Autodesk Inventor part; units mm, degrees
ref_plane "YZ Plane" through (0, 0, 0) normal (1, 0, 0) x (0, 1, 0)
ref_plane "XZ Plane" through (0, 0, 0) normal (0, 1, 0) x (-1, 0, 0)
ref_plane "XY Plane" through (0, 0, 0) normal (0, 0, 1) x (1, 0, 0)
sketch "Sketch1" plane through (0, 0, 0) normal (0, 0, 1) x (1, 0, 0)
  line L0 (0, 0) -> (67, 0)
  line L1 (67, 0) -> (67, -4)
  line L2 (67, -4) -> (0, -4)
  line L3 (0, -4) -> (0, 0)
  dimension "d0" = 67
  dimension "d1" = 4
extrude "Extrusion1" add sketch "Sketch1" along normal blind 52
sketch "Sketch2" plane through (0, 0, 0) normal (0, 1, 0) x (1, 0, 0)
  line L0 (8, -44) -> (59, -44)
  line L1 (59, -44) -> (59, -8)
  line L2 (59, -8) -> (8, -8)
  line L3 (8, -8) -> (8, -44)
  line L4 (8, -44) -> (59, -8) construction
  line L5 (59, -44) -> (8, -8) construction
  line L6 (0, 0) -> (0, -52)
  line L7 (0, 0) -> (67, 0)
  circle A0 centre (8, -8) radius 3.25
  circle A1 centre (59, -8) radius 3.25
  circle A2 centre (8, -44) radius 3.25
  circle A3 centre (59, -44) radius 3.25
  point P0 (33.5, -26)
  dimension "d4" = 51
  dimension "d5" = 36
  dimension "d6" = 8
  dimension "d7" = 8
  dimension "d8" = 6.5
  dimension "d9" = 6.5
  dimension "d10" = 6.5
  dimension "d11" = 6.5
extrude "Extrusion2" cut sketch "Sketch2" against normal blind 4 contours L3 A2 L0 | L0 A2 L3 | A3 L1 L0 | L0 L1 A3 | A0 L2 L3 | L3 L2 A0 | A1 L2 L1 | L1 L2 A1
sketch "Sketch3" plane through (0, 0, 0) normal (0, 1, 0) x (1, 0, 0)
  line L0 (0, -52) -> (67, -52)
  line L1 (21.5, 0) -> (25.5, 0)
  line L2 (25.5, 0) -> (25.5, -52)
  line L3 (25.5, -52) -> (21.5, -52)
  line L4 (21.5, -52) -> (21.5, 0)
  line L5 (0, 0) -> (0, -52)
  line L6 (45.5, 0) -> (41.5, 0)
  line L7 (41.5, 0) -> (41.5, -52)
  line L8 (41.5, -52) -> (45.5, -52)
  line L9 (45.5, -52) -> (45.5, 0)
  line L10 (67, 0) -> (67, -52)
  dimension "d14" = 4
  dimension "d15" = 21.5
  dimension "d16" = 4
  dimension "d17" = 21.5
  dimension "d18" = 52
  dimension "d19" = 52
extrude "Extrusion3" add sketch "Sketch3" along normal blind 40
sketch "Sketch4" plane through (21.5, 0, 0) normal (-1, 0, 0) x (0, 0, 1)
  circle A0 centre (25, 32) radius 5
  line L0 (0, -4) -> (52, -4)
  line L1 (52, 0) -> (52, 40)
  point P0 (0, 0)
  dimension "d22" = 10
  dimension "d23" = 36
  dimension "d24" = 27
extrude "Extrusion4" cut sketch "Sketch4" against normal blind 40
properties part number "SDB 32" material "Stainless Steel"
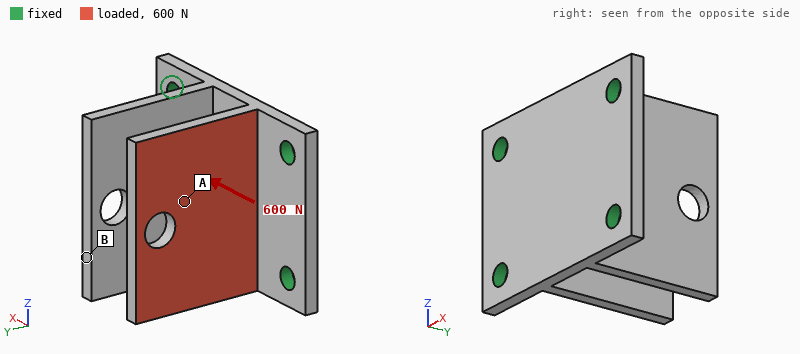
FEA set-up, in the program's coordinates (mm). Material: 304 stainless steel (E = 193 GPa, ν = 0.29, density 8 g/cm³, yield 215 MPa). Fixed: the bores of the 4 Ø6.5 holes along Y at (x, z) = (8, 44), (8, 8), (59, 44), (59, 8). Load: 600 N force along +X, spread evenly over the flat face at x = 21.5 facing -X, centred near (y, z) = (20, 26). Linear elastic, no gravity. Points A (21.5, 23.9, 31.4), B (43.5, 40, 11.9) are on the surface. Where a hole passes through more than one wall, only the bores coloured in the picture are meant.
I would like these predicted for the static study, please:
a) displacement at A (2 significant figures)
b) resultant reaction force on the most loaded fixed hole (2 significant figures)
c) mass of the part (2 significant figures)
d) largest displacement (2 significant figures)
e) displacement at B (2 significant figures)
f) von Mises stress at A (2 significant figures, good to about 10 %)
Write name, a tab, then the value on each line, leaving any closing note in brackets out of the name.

displacement at A	0.066 mm
resultant reaction force on the most loaded fixed hole	250 N
mass of the part	240 g
largest displacement	0.13 mm
displacement at B	0.020 mm
von Mises stress at A	13 MPa
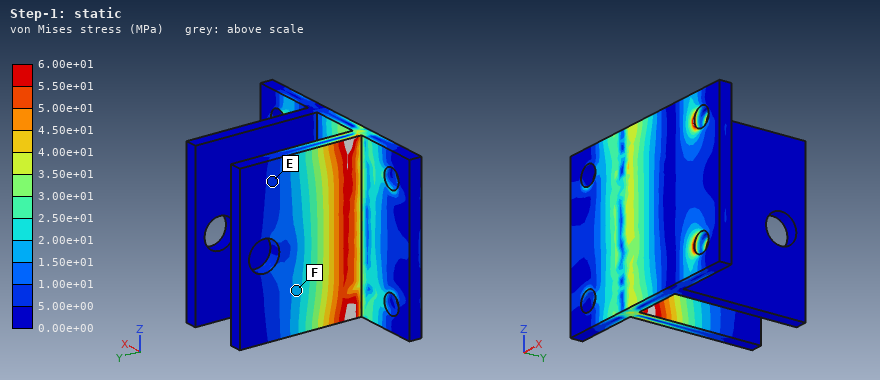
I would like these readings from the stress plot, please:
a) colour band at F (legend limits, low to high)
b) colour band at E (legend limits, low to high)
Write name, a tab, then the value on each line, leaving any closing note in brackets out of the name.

colour band at F	1.50e+01 to 2.00e+01 MPa
colour band at E	5.00e+00 to 1.00e+01 MPa
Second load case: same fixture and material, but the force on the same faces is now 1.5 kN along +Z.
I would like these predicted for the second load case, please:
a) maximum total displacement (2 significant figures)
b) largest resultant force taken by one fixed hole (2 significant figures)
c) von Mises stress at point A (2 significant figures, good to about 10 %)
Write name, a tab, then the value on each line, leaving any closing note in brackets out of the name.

maximum total displacement	43 µm
largest resultant force taken by one fixed hole	870 N
von Mises stress at point A	16 MPa
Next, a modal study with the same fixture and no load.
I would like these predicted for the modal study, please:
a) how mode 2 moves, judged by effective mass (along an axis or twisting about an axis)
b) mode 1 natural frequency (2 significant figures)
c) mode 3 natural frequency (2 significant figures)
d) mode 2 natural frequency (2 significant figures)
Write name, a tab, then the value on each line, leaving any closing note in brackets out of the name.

how mode 2 moves, judged by effective mass	along X
mode 1 natural frequency	1600 Hz
mode 3 natural frequency	3200 Hz
mode 2 natural frequency	1900 Hz
